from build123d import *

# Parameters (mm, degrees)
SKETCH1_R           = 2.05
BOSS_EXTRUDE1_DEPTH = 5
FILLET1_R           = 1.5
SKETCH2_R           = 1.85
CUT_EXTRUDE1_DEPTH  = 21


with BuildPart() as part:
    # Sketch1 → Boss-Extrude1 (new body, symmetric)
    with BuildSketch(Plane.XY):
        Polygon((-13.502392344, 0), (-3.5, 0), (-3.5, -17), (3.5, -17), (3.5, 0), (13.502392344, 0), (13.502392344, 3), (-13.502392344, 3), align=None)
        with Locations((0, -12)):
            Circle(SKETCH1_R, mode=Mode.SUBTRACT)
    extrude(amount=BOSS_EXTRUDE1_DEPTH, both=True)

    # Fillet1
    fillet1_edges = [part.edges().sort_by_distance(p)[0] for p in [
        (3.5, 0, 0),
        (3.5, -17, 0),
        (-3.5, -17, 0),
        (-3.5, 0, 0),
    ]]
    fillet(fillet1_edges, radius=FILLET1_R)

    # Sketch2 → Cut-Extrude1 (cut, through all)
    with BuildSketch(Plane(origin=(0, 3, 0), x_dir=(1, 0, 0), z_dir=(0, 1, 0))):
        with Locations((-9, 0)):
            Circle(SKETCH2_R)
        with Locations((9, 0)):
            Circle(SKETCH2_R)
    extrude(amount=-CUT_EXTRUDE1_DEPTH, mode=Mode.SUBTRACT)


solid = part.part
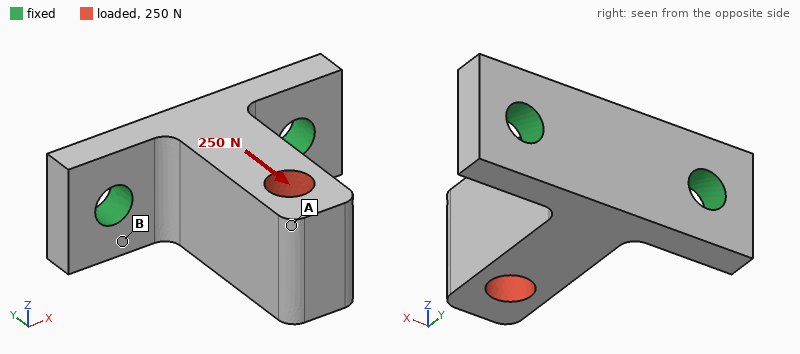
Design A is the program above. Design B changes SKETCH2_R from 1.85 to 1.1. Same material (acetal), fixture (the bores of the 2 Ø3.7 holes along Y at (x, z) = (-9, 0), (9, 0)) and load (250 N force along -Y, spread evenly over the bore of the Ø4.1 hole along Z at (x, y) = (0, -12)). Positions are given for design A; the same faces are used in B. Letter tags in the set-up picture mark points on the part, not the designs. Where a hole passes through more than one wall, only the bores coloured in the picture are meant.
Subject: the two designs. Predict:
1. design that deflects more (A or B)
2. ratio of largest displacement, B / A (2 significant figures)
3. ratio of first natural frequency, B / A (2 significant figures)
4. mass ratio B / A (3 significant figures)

B
1.3
0.86
1.02
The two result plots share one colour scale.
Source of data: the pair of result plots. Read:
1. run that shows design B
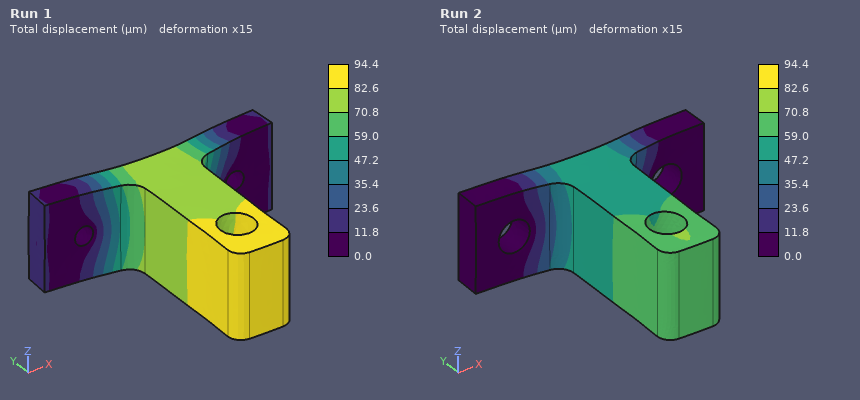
Run 1
